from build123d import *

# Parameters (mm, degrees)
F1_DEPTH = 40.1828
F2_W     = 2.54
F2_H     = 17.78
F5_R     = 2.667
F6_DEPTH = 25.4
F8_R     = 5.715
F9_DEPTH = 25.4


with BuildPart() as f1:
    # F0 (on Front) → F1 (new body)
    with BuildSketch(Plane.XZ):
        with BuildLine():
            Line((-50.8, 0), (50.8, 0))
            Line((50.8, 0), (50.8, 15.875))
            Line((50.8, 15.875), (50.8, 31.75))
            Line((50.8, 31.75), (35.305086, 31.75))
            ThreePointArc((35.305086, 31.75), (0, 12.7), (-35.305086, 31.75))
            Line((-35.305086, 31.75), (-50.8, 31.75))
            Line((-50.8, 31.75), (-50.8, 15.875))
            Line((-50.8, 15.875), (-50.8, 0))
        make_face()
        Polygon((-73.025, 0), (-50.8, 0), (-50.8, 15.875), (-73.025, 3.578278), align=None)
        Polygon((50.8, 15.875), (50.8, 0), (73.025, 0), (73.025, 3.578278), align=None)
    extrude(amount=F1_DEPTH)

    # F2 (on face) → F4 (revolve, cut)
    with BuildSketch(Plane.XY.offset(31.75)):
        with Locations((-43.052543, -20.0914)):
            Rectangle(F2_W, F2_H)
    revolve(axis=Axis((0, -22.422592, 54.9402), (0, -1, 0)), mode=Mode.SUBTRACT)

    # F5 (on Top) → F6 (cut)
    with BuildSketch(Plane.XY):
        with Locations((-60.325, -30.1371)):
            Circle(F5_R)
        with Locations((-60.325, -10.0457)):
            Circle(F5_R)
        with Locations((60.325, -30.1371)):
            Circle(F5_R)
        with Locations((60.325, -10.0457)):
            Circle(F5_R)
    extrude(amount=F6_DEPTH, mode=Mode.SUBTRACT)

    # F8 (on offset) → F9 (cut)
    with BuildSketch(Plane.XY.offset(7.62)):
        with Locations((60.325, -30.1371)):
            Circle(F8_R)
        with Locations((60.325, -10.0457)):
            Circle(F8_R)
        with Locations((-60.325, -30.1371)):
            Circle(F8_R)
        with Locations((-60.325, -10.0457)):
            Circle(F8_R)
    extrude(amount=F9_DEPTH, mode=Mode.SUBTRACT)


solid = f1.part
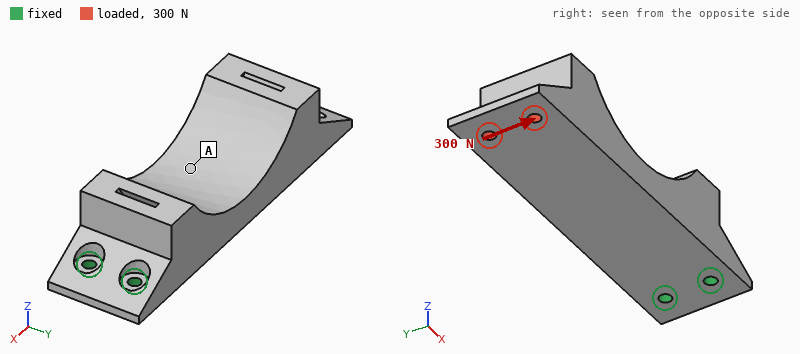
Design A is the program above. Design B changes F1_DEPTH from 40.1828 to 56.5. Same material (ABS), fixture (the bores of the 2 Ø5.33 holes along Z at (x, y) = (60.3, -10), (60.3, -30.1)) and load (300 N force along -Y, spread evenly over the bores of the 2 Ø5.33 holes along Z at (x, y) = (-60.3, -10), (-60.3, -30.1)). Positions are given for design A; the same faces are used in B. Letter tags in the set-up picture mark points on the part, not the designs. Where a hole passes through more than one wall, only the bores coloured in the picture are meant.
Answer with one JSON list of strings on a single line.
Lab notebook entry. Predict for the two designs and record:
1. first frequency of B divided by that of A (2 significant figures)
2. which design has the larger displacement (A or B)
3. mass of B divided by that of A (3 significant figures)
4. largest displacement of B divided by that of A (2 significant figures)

["0.89", "A", "1.43", "0.73"]
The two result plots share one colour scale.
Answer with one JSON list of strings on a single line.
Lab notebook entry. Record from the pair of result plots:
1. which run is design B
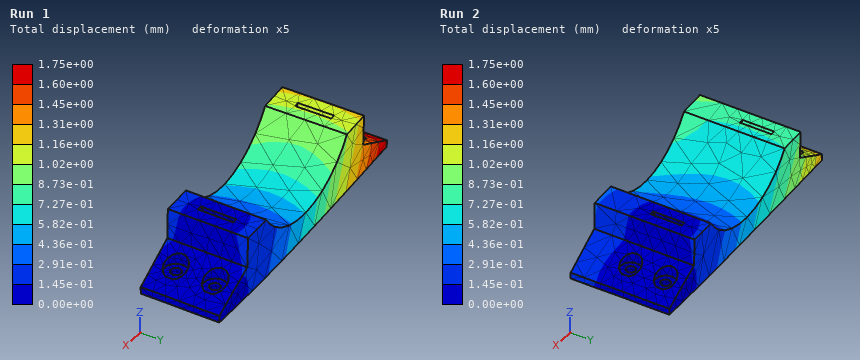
["Run 2"]
